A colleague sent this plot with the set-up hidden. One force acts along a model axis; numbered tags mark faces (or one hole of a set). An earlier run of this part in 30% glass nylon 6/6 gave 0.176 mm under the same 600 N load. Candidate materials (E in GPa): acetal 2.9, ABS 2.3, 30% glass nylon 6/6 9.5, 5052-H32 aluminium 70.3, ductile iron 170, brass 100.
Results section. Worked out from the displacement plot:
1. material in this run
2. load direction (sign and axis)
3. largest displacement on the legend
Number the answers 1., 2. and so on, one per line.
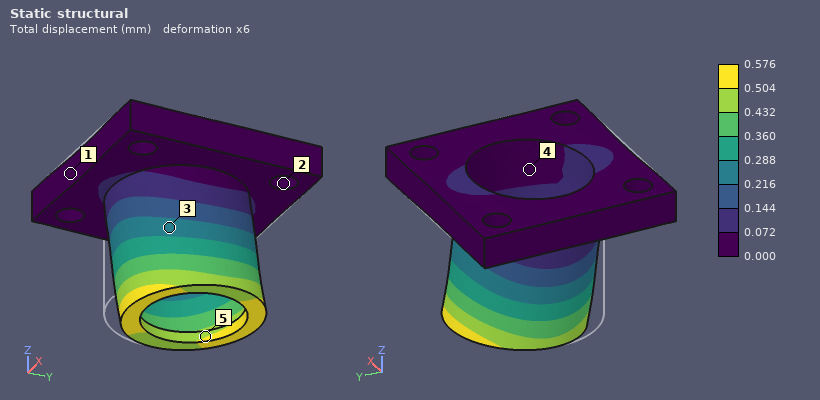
1. acetal
2. +Y
3. 0.576 mm
